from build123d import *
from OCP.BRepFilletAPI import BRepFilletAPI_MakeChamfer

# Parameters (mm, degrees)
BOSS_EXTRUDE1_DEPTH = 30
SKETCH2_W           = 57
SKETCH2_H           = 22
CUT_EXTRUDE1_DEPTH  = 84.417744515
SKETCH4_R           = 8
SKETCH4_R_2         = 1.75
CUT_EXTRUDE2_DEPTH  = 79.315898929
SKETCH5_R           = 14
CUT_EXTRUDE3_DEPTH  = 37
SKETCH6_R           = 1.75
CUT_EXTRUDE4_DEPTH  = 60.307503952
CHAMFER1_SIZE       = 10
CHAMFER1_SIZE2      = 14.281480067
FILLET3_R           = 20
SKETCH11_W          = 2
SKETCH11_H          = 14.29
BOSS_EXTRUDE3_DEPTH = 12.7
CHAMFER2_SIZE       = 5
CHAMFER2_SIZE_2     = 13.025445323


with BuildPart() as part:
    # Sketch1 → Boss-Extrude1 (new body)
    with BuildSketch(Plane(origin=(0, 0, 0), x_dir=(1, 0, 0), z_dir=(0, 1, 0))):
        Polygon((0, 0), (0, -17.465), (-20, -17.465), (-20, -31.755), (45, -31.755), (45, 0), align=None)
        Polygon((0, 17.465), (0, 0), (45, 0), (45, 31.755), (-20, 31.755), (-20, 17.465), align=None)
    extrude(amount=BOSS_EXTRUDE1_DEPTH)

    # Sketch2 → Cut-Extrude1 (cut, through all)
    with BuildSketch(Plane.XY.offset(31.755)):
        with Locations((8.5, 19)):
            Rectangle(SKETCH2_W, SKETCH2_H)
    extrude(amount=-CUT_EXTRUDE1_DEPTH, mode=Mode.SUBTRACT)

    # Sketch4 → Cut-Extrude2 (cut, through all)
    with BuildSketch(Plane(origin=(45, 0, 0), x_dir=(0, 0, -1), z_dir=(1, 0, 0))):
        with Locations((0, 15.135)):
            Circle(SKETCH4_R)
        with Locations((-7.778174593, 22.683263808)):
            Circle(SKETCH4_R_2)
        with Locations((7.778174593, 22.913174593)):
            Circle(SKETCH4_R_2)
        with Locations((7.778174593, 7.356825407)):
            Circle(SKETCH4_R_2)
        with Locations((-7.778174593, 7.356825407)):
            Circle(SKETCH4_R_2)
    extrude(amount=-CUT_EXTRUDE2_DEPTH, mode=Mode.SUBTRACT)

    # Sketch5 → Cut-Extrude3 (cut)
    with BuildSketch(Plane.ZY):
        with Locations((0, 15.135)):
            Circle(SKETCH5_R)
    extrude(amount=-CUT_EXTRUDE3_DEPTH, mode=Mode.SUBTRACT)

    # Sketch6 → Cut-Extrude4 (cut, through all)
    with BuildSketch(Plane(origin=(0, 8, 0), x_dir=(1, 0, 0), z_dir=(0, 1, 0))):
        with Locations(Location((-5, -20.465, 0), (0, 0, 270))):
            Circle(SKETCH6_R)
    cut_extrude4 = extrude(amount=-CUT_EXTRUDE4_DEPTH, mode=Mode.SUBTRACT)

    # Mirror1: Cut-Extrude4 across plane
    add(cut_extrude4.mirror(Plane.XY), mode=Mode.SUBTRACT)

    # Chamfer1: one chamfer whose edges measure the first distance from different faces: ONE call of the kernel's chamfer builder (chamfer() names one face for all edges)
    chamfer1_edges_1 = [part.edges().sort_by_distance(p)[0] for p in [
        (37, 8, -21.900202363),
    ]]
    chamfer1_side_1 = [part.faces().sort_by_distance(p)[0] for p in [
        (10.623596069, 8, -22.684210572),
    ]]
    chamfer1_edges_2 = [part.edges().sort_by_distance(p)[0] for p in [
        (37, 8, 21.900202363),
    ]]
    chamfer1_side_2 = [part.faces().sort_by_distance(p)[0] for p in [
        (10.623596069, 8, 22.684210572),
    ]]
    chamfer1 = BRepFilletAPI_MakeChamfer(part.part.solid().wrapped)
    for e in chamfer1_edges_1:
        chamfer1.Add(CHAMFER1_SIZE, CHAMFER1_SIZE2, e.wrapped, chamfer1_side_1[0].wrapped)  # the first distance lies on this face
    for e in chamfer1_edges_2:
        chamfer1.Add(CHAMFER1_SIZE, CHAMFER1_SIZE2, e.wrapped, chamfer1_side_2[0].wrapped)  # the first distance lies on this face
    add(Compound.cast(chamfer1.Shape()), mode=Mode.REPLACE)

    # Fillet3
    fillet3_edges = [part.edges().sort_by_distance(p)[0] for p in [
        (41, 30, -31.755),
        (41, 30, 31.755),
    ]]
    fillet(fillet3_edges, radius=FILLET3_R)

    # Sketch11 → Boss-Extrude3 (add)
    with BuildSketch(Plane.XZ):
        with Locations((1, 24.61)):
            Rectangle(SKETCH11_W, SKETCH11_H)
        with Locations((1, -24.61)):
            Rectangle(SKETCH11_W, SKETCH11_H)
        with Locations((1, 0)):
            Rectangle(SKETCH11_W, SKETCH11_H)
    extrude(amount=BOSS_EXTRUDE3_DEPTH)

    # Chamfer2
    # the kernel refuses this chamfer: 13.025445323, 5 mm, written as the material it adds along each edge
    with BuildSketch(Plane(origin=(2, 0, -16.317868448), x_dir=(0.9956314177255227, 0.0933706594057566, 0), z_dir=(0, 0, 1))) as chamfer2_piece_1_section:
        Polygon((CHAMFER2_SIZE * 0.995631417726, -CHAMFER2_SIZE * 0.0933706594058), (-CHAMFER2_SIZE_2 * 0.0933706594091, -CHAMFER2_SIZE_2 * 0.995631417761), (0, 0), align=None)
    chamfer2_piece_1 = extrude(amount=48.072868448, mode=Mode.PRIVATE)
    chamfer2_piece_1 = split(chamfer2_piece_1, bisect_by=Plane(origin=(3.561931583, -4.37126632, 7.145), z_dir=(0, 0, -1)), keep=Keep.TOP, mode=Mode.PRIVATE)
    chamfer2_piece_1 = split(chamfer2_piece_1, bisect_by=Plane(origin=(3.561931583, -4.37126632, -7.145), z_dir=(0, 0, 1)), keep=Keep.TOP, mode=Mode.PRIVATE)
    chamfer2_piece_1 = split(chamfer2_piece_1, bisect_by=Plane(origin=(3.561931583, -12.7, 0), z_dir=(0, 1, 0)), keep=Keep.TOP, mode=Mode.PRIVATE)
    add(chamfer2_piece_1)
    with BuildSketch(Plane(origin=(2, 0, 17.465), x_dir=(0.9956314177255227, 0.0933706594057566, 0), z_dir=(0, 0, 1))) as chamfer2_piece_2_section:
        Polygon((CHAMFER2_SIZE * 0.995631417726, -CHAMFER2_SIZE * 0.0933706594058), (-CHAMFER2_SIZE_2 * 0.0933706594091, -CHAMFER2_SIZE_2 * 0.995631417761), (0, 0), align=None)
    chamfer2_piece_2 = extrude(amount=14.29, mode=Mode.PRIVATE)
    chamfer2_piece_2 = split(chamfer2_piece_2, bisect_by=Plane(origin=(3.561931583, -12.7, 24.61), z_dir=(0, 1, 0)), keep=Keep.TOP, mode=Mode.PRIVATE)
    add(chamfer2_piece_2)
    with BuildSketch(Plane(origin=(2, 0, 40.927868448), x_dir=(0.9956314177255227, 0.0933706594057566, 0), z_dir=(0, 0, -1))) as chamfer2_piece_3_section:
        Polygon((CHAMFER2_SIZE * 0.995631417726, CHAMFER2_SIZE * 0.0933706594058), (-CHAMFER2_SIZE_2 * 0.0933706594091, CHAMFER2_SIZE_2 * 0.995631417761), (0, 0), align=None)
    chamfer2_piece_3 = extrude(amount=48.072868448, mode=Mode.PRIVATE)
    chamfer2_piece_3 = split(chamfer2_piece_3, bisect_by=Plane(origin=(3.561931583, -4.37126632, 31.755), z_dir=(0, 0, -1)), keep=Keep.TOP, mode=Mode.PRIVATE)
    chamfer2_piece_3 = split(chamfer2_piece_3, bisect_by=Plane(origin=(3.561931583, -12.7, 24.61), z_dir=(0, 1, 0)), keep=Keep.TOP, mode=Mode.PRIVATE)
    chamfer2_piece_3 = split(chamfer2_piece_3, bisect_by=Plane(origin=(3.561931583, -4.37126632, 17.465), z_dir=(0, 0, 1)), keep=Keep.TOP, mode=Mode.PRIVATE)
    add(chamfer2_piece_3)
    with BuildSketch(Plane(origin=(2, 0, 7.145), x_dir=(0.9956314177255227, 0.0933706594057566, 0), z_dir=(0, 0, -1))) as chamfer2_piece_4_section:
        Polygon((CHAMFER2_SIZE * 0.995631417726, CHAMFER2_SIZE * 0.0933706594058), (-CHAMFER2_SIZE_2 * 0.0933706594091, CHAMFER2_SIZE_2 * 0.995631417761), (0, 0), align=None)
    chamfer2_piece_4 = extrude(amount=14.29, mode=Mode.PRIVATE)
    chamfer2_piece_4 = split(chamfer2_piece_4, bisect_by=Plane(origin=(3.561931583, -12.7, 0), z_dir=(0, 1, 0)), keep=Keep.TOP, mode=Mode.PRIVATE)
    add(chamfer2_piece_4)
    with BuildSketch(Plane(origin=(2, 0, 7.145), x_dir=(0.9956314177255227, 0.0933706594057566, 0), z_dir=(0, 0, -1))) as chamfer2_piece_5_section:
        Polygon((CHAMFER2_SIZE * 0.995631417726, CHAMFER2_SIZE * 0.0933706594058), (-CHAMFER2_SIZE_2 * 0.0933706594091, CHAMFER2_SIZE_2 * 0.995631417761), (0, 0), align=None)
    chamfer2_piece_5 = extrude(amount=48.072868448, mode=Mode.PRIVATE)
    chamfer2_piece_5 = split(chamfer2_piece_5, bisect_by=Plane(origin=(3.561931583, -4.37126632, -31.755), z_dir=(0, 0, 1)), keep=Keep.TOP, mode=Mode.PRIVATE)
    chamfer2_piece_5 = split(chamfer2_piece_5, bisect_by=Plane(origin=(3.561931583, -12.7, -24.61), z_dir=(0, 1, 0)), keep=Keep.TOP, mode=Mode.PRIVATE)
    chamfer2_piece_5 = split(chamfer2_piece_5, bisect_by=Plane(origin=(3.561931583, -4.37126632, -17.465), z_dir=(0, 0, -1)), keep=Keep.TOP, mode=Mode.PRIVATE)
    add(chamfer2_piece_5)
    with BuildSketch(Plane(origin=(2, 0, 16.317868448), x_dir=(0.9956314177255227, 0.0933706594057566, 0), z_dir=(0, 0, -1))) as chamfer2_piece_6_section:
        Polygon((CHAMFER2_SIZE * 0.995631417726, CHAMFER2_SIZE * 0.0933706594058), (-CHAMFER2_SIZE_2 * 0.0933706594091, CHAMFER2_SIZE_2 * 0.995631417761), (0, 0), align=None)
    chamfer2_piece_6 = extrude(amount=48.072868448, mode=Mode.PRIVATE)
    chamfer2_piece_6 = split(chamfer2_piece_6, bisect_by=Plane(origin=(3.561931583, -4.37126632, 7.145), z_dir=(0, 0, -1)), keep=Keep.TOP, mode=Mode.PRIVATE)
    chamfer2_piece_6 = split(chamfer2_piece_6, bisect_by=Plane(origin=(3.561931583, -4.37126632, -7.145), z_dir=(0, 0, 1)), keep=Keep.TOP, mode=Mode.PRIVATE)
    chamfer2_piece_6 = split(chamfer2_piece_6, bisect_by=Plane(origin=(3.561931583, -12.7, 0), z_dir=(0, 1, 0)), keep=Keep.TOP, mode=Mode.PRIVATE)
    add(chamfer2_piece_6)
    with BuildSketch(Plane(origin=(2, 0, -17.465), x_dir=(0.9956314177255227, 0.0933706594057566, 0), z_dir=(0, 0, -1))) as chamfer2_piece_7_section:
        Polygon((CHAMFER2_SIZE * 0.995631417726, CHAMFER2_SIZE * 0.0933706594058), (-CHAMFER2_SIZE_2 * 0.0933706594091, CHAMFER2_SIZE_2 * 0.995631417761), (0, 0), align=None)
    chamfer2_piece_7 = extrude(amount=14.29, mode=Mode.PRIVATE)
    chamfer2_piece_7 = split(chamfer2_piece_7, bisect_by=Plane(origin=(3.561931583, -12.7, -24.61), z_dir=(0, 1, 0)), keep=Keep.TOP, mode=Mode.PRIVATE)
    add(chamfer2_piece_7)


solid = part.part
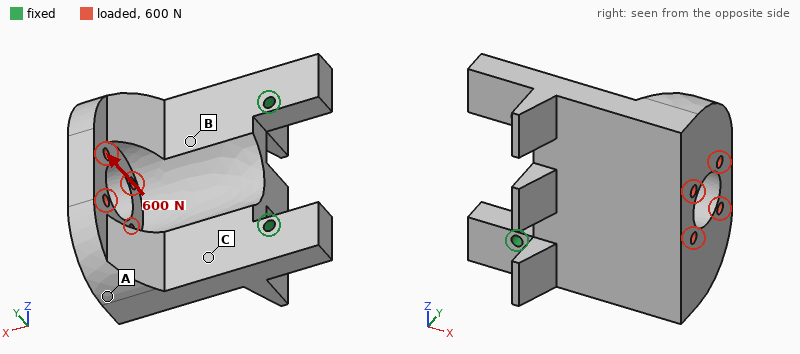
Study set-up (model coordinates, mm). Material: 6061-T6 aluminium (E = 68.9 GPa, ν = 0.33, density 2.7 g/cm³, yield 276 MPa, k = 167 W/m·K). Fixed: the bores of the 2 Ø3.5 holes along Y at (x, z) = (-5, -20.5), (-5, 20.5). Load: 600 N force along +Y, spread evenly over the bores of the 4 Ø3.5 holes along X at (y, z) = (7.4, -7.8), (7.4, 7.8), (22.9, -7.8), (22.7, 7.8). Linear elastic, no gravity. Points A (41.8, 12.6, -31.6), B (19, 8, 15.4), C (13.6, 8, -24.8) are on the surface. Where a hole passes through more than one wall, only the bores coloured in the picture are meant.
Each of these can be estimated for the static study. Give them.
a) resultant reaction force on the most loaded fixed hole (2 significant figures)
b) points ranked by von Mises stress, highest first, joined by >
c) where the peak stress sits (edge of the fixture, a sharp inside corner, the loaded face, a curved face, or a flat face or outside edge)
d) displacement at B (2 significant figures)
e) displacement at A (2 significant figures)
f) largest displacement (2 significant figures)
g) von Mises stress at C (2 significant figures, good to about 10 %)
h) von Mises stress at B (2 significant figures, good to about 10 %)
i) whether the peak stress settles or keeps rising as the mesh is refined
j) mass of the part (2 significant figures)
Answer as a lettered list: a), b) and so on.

a) 320 N
b) C > B > A
c) edge of the fixture
d) 0.078 mm
e) 0.20 mm
f) 0.26 mm
g) 35 MPa
h) 27 MPa
i) keeps rising
j) 97 g
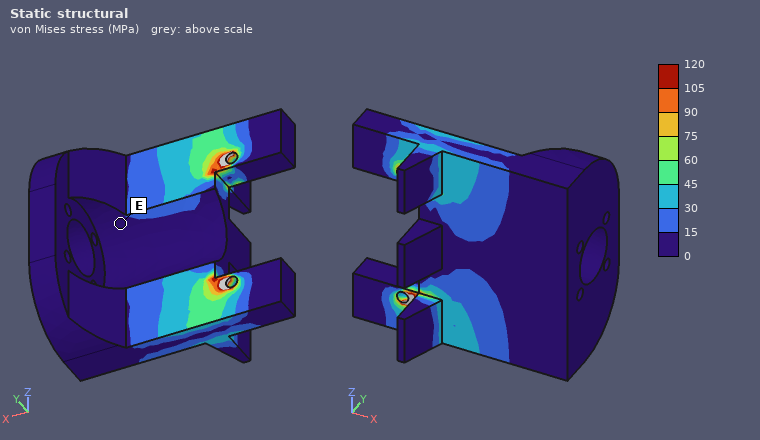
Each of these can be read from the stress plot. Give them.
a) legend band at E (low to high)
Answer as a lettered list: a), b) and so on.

a) 0 to 15 MPa
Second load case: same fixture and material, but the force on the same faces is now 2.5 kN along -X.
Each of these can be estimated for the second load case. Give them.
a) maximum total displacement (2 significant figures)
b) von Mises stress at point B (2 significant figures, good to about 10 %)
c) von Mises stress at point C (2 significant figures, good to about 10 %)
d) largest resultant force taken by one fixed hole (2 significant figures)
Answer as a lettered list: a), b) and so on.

a) 0.39 mm
b) 68 MPa
c) 66 MPa
d) 1.3 kN
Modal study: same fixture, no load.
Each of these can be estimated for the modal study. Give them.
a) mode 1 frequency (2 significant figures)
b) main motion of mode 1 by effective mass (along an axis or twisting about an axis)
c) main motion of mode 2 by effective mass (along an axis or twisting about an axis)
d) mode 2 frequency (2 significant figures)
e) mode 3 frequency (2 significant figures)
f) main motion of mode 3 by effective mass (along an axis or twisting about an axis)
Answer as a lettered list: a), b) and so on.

a) 1200 Hz
b) along Y
c) along Z
d) 2800 Hz
e) 5200 Hz
f) along Z
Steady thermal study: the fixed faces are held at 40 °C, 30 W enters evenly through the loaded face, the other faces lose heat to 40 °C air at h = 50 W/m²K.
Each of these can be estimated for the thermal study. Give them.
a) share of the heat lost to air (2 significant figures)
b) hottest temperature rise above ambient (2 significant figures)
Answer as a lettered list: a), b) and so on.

a) 26 %
b) 24 K
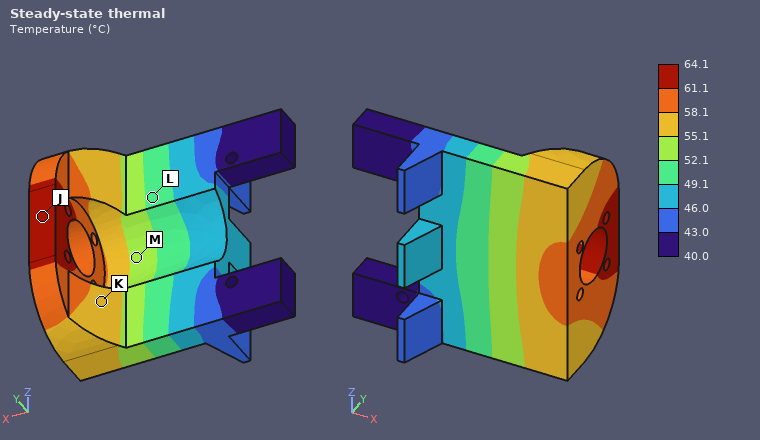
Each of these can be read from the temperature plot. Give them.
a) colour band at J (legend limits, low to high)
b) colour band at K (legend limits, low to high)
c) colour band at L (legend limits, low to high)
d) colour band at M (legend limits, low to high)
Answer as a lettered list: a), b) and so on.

a) 61.1 to 64.1 °C
b) 55.1 to 58.1 °C
c) 49.1 to 52.1 °C
d) 52.1 to 55.1 °C
